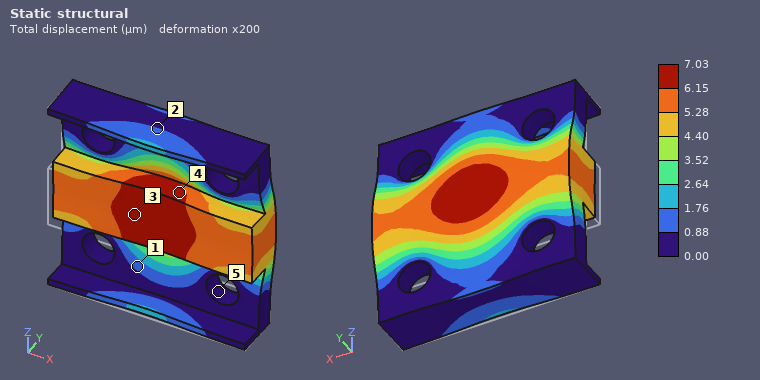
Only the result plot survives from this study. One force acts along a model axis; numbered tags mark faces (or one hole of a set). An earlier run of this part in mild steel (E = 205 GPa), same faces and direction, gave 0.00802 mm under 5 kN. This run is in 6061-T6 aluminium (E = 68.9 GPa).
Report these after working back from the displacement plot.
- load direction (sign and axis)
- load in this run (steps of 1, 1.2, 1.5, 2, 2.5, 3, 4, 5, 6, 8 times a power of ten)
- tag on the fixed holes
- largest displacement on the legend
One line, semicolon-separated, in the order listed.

+Y; 1.5 kN; 5; 7.03 µm
